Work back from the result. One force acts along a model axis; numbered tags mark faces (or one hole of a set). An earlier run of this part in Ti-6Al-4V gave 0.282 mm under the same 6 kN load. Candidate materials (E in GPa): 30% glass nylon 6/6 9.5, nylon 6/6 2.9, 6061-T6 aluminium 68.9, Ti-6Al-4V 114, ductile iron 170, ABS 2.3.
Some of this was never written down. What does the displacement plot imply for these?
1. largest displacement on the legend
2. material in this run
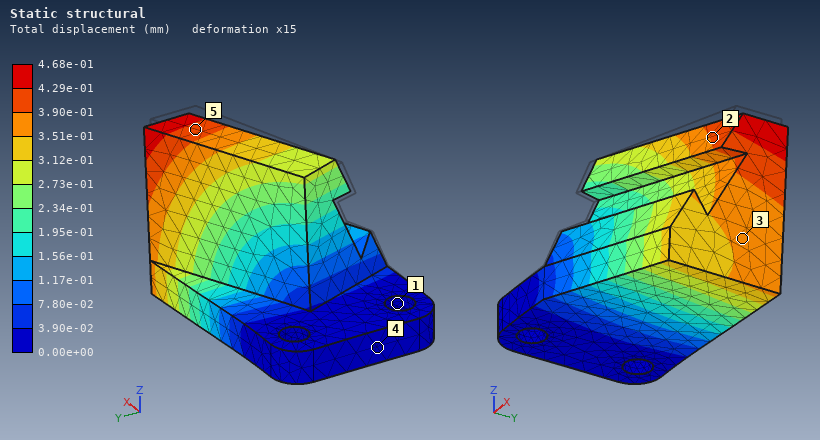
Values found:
4.68e-01 mm
6061-T6 aluminium
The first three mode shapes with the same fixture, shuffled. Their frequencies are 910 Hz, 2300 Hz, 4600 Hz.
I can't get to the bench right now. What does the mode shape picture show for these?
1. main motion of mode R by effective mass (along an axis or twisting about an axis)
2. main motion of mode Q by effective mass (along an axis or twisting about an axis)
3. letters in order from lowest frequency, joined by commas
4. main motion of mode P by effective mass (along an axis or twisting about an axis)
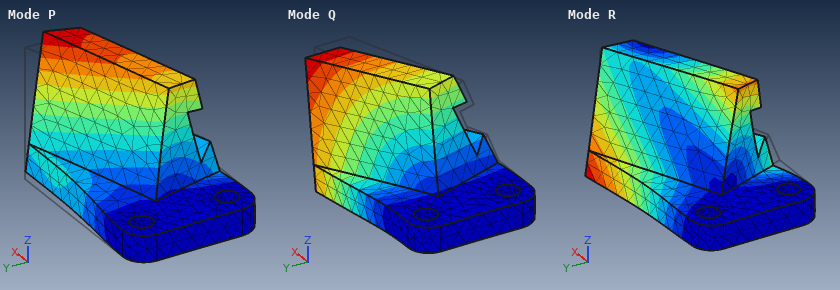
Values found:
along Y
along Z
Q, P, R
along Y
